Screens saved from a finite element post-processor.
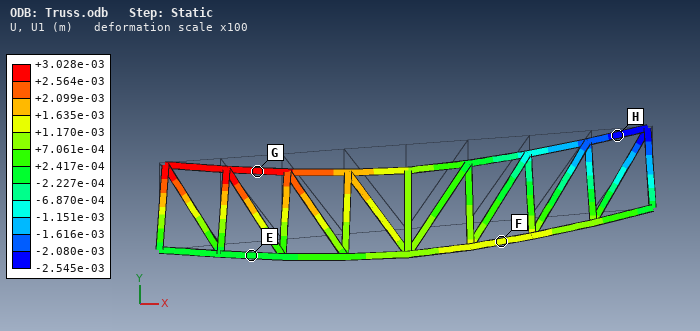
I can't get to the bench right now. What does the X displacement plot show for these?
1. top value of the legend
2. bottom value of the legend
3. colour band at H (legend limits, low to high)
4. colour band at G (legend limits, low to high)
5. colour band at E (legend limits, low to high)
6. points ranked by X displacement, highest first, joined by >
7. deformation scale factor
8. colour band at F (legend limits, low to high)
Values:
+3.028e-03 m
-2.545e-03 m
-2.545e-03 to -2.080e-03 m
+2.564e-03 to +3.028e-03 m
-2.227e-04 to +2.417e-04 m
G > F > E > H
100
+1.170e-03 to +1.635e-03 m
